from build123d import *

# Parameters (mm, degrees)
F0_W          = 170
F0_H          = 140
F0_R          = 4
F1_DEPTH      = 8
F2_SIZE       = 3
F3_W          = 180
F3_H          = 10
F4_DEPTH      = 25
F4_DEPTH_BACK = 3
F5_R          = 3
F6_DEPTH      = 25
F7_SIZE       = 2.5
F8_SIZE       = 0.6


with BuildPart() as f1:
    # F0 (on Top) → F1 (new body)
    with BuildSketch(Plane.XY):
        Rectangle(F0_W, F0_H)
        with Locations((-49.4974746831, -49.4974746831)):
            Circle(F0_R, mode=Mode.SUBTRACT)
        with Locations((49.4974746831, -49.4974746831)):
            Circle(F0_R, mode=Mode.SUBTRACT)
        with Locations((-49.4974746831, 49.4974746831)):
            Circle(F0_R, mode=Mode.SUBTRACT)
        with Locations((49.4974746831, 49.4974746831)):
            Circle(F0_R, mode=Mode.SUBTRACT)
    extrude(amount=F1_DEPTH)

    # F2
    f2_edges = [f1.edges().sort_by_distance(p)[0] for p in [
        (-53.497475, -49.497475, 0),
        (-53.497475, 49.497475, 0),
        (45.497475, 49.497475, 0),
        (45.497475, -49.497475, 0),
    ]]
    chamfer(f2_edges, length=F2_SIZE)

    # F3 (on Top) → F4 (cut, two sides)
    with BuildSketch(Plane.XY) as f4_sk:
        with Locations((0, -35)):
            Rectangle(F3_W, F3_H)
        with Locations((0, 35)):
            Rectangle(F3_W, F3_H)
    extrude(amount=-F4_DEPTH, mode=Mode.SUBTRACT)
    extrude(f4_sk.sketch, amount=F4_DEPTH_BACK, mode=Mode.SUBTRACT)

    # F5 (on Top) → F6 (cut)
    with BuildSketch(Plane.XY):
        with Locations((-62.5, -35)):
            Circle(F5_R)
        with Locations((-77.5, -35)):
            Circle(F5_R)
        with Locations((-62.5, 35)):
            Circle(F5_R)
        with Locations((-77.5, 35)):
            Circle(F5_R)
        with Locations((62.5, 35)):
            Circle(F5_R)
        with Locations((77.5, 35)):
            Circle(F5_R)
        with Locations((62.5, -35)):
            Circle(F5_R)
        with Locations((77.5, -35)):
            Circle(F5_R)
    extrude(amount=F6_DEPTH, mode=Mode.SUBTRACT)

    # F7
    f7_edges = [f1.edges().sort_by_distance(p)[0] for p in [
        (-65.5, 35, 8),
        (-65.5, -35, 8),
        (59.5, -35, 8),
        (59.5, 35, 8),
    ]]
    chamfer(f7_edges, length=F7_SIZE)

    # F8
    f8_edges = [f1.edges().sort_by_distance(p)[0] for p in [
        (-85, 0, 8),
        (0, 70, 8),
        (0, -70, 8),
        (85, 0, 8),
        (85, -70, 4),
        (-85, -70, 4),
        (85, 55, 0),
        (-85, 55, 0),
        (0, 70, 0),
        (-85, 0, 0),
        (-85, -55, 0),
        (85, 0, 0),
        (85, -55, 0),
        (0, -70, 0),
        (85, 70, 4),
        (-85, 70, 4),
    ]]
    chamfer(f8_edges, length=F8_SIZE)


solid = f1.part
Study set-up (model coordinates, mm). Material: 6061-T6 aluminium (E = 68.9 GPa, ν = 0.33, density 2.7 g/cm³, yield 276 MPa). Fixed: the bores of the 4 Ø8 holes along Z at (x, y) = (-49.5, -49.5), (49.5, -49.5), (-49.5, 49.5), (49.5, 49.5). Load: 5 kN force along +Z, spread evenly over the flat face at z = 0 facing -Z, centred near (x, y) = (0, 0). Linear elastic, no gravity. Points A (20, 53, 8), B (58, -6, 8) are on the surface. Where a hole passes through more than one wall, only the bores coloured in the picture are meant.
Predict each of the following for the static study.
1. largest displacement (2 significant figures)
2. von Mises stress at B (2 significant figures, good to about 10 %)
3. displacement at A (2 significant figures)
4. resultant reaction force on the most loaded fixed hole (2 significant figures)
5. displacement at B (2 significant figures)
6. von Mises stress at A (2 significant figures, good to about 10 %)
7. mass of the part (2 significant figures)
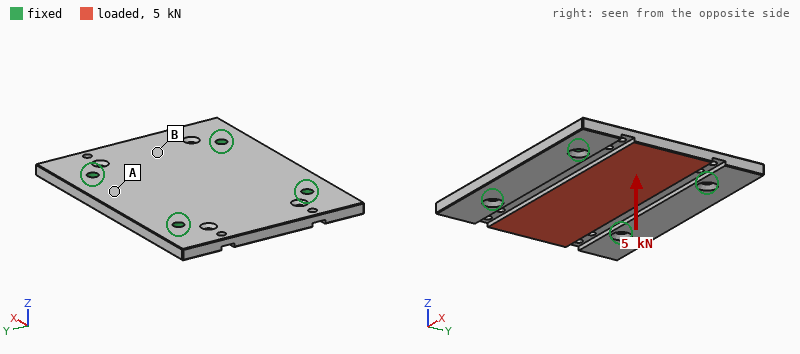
99 µm
24 MPa
16 µm
1.5 kN
80 µm
8.6 MPa
480 g
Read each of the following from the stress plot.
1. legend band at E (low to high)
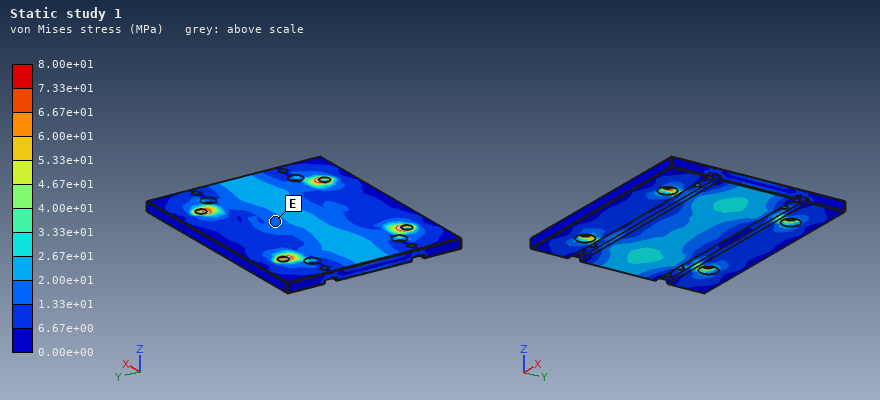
1.33e+01 to 2.00e+01 MPa
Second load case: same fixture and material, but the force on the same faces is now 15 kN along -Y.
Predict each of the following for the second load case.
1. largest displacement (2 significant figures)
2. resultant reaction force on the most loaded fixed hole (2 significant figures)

18 µm
3.8 kN
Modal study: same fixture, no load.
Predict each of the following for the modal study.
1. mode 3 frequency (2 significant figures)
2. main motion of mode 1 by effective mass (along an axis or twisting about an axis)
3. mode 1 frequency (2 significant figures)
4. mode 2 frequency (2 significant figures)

2700 Hz
along Z
2600 Hz
2700 Hz
